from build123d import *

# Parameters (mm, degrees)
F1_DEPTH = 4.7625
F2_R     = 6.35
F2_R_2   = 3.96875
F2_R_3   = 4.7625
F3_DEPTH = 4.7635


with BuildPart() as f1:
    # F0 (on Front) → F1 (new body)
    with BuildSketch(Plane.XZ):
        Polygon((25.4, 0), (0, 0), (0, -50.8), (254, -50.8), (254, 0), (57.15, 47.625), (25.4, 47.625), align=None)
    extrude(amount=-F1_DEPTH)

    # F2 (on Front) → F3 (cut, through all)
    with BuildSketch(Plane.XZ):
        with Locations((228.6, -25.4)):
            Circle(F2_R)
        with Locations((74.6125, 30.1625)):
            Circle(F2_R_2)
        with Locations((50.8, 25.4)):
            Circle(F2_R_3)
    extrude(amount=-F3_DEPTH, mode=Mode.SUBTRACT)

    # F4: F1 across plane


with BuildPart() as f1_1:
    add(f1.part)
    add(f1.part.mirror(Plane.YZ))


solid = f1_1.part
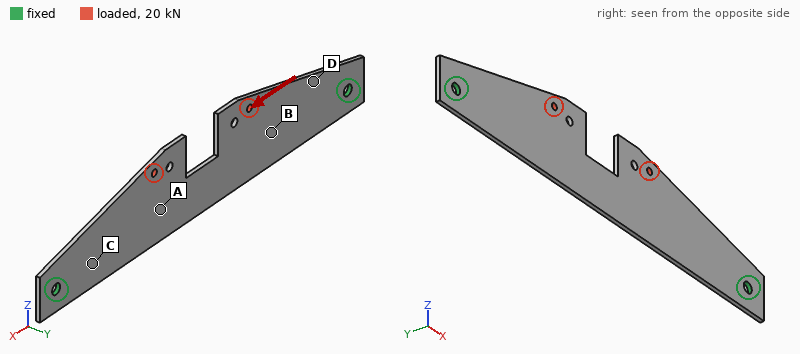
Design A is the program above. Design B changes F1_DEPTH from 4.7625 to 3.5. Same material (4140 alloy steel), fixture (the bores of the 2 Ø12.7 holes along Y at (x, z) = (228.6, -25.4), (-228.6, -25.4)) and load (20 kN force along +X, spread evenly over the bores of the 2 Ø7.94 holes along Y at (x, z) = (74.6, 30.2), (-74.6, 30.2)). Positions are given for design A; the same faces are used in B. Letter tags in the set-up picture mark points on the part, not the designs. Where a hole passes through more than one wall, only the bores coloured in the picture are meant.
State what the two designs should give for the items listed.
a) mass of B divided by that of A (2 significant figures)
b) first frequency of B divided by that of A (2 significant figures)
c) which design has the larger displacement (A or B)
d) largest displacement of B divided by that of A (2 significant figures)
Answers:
0.73
0.74
B
1.4
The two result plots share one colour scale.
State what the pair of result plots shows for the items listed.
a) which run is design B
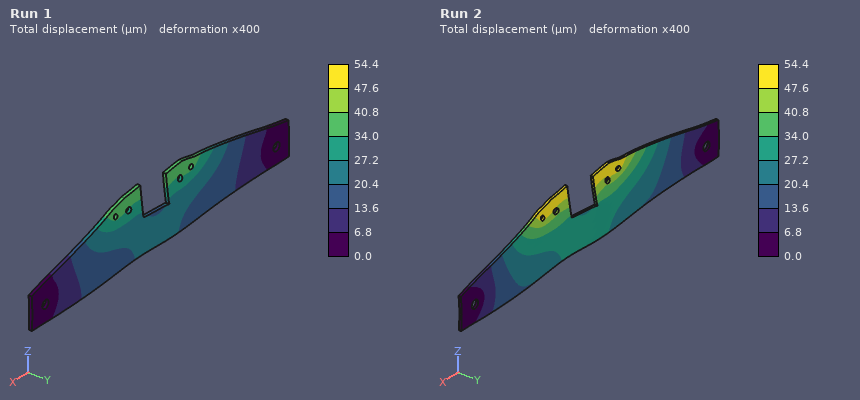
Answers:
Run 2
